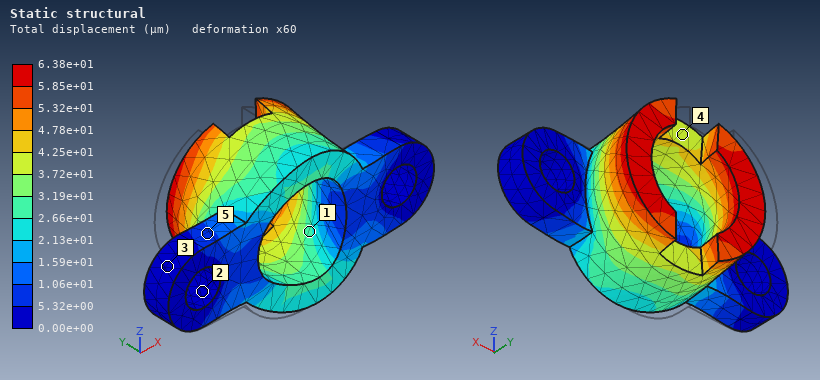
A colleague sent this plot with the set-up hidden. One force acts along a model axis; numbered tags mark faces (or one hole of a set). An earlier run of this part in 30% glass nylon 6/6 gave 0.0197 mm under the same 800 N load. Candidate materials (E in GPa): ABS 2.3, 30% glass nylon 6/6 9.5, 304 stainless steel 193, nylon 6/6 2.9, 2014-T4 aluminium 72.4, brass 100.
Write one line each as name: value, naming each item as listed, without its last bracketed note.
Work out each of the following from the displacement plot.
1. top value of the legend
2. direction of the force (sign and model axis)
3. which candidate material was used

top value of the legend: 6.38e+01 µm
direction of the force: +X
which candidate material was used: nylon 6/6
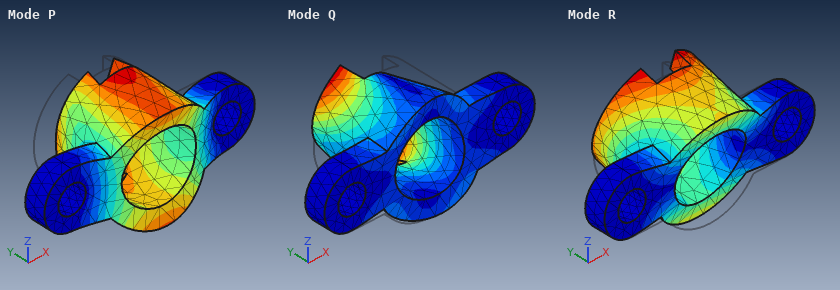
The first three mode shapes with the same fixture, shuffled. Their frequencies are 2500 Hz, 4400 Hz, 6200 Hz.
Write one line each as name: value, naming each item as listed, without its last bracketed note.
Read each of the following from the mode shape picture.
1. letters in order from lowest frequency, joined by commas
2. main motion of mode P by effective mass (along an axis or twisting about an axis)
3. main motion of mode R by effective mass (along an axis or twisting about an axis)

letters in order from lowest frequency, joined by commas: R, P, Q
main motion of mode P by effective mass: along Y
main motion of mode R by effective mass: along Z
